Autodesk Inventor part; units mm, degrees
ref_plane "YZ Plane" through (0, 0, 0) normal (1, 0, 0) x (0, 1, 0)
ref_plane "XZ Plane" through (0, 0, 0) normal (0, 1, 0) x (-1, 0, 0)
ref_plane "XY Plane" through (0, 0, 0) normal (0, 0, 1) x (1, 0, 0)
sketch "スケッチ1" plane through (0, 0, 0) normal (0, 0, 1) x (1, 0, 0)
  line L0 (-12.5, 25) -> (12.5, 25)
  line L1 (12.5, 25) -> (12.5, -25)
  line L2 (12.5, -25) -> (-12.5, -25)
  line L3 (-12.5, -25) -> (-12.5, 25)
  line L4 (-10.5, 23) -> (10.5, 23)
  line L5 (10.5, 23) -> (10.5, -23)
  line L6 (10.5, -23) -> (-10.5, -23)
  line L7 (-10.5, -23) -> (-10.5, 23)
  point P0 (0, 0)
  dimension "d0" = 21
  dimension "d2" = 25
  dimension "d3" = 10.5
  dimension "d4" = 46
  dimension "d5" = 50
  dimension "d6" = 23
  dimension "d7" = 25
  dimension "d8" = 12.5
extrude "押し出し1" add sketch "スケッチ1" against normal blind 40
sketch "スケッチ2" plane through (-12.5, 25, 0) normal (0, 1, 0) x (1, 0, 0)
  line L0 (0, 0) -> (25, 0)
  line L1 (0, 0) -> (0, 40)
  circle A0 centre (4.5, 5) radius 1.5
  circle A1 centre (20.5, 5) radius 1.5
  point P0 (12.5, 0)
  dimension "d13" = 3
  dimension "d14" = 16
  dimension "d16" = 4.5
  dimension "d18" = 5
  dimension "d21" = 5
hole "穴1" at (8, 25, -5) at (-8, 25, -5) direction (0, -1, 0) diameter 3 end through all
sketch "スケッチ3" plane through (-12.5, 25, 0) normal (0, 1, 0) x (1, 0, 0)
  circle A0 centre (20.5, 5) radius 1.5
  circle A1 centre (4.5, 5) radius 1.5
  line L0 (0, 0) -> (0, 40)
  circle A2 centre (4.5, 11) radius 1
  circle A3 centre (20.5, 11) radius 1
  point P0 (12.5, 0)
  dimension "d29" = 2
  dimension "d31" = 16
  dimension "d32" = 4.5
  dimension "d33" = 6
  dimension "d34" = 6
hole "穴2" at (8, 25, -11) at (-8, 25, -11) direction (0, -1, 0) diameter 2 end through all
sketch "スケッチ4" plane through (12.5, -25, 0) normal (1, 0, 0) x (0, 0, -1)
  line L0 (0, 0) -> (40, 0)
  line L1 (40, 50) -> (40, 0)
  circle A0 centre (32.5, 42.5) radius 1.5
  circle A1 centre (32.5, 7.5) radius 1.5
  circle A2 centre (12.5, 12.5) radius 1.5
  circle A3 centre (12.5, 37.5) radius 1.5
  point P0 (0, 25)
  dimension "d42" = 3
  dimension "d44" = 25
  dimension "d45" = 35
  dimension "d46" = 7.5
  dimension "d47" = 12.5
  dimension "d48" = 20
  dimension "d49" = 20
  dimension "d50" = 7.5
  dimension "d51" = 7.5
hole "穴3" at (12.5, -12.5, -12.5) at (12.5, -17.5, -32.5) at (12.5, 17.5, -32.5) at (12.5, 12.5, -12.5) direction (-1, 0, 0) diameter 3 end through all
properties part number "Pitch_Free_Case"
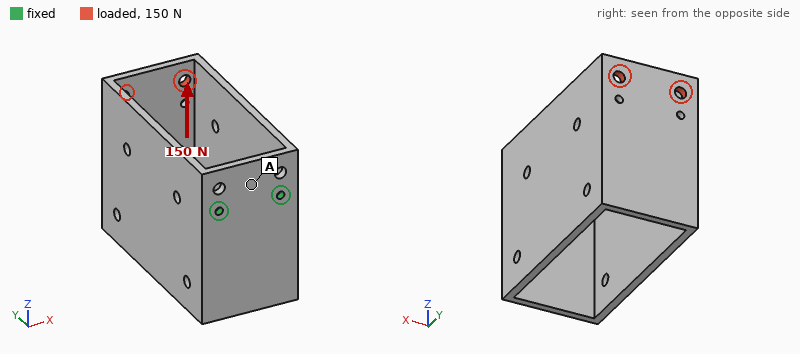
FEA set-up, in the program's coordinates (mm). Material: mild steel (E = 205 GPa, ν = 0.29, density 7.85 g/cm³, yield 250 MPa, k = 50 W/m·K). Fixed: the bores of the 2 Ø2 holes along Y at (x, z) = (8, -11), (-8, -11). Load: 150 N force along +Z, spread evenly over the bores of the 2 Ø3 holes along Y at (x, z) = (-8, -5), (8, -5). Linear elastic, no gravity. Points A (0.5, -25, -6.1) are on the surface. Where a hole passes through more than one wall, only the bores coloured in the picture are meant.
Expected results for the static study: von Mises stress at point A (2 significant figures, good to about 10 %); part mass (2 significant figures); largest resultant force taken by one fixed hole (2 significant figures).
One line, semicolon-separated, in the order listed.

32 MPa; 88 g; 75 N
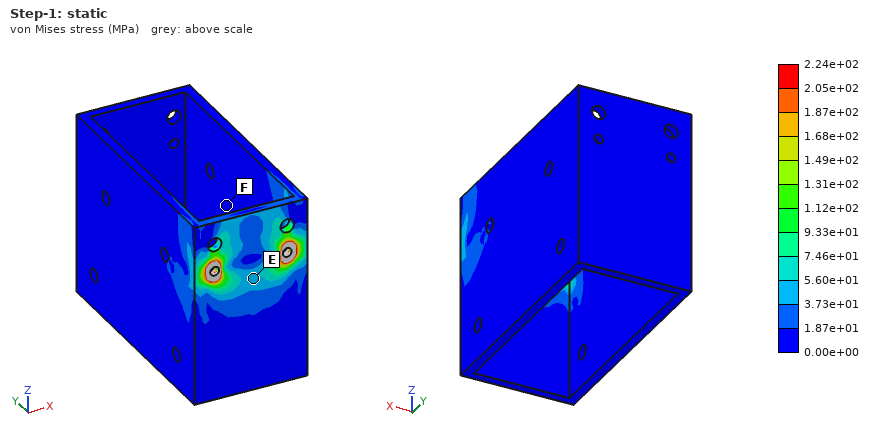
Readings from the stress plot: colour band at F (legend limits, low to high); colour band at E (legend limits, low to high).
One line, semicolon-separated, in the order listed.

0.00e+00 to 1.87e+01 MPa; 3.73e+01 to 5.60e+01 MPa
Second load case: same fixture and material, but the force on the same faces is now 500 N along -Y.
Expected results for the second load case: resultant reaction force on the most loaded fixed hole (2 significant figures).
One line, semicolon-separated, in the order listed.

250 N
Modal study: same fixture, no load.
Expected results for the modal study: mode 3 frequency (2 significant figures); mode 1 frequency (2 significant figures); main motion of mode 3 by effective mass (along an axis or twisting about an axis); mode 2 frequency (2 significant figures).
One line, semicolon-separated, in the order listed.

1800 Hz; 700 Hz; twisting about Y; 700 Hz
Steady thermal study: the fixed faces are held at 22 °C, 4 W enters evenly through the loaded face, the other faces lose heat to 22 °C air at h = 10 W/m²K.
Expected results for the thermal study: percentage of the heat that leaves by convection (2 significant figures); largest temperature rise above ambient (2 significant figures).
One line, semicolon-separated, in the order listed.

41 %; 35 K
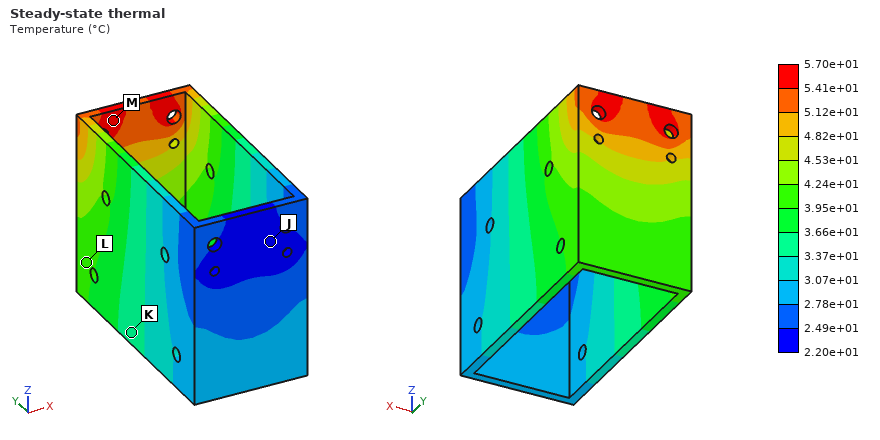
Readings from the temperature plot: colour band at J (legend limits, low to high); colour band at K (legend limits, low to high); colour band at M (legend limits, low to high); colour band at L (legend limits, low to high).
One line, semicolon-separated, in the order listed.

2.20e+01 to 2.49e+01 °C; 3.37e+01 to 3.66e+01 °C; 5.41e+01 to 5.70e+01 °C; 3.95e+01 to 4.24e+01 °C
